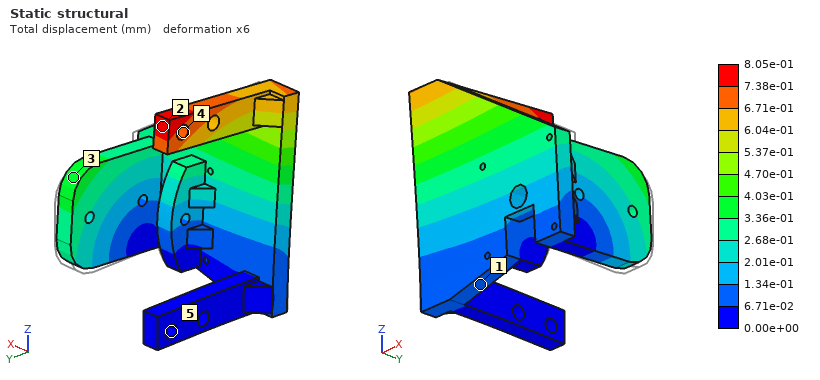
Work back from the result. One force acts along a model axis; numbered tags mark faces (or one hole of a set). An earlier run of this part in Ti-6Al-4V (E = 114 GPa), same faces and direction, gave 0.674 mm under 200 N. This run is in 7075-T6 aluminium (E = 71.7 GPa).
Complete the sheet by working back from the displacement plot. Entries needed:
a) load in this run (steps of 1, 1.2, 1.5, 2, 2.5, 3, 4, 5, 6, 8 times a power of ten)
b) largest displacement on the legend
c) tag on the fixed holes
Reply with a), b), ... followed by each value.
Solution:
a) 150 N
b) 8.05e-01 mm
c) 5
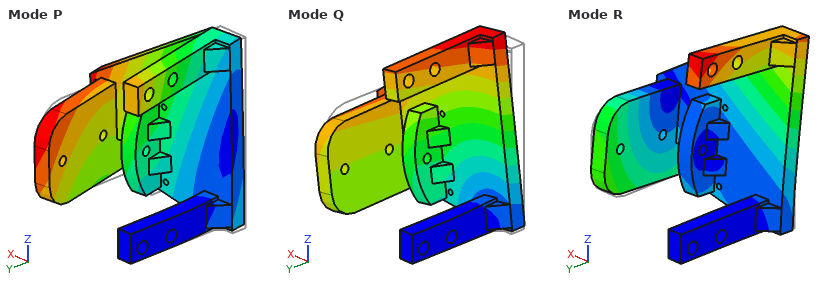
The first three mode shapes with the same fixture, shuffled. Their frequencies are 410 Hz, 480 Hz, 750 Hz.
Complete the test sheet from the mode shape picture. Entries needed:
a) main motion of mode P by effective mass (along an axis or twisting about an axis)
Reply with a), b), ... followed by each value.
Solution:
a) along Y
